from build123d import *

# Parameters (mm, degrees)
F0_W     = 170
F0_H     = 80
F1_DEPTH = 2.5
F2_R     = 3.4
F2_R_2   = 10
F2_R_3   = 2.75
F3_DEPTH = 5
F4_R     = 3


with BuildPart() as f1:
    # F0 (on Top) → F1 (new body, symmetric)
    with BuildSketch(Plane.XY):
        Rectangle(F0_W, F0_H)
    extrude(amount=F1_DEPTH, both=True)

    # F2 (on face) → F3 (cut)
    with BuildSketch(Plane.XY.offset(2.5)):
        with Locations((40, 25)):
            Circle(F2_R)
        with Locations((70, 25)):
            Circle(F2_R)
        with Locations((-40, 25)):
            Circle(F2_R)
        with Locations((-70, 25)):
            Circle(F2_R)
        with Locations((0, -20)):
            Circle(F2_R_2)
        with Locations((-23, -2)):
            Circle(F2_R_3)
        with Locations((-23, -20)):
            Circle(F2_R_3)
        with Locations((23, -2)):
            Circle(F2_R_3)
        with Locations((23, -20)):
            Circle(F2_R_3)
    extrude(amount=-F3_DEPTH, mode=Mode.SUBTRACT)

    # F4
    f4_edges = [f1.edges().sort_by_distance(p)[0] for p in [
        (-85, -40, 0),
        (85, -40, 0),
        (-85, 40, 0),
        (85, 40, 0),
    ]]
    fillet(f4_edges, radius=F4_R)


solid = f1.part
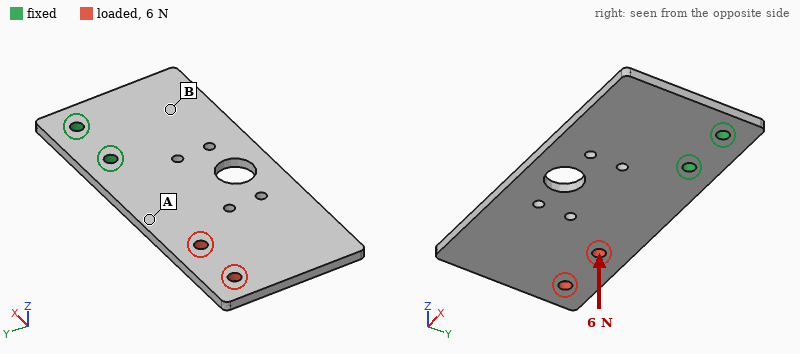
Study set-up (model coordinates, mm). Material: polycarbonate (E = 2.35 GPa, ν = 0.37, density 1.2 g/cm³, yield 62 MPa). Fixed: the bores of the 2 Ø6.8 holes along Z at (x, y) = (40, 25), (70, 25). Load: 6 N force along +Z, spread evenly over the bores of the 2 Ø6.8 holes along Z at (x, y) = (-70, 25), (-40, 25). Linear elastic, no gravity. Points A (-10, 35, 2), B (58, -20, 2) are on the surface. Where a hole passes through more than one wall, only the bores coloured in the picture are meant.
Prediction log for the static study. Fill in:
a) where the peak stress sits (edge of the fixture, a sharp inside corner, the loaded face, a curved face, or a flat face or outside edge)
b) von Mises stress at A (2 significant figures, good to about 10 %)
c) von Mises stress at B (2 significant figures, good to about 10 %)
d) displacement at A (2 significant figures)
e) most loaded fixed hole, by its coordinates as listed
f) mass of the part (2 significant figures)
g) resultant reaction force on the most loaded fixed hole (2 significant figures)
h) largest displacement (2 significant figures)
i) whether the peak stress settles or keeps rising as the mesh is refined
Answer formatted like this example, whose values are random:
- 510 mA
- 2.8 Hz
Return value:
- edge of the fixture
- 1.1 MPa
- 0.45 MPa
- 0.42 mm
- (40, 25)
- 78 g
- 14 N
- 1.7 mm
- keeps rising
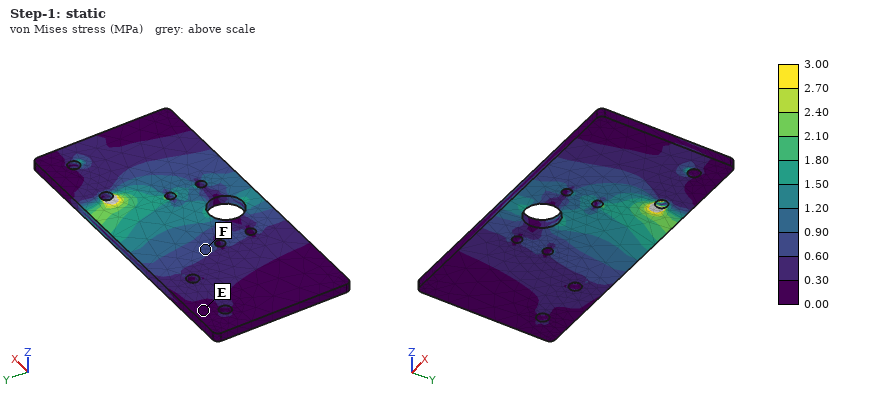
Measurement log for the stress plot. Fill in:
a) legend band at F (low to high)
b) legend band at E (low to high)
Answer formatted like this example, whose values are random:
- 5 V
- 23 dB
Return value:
- 0.60 to 0.90 MPa
- 0.00 to 0.30 MPa
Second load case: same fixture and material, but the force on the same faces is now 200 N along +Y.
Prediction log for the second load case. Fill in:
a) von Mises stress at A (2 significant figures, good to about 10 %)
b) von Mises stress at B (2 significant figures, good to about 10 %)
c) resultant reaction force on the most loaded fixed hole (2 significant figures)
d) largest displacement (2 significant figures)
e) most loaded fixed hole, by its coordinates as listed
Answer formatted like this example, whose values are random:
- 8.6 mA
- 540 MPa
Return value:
- 1.4 MPa
- 2.0 MPa
- 730 N
- 0.86 mm
- (40, 25)
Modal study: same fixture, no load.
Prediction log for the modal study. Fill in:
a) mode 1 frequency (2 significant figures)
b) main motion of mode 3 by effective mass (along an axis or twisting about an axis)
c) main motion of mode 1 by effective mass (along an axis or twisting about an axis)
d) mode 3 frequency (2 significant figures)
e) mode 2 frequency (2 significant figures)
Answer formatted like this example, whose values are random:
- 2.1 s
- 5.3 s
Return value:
- 63 Hz
- along Z
- along Z
- 330 Hz
- 180 Hz
